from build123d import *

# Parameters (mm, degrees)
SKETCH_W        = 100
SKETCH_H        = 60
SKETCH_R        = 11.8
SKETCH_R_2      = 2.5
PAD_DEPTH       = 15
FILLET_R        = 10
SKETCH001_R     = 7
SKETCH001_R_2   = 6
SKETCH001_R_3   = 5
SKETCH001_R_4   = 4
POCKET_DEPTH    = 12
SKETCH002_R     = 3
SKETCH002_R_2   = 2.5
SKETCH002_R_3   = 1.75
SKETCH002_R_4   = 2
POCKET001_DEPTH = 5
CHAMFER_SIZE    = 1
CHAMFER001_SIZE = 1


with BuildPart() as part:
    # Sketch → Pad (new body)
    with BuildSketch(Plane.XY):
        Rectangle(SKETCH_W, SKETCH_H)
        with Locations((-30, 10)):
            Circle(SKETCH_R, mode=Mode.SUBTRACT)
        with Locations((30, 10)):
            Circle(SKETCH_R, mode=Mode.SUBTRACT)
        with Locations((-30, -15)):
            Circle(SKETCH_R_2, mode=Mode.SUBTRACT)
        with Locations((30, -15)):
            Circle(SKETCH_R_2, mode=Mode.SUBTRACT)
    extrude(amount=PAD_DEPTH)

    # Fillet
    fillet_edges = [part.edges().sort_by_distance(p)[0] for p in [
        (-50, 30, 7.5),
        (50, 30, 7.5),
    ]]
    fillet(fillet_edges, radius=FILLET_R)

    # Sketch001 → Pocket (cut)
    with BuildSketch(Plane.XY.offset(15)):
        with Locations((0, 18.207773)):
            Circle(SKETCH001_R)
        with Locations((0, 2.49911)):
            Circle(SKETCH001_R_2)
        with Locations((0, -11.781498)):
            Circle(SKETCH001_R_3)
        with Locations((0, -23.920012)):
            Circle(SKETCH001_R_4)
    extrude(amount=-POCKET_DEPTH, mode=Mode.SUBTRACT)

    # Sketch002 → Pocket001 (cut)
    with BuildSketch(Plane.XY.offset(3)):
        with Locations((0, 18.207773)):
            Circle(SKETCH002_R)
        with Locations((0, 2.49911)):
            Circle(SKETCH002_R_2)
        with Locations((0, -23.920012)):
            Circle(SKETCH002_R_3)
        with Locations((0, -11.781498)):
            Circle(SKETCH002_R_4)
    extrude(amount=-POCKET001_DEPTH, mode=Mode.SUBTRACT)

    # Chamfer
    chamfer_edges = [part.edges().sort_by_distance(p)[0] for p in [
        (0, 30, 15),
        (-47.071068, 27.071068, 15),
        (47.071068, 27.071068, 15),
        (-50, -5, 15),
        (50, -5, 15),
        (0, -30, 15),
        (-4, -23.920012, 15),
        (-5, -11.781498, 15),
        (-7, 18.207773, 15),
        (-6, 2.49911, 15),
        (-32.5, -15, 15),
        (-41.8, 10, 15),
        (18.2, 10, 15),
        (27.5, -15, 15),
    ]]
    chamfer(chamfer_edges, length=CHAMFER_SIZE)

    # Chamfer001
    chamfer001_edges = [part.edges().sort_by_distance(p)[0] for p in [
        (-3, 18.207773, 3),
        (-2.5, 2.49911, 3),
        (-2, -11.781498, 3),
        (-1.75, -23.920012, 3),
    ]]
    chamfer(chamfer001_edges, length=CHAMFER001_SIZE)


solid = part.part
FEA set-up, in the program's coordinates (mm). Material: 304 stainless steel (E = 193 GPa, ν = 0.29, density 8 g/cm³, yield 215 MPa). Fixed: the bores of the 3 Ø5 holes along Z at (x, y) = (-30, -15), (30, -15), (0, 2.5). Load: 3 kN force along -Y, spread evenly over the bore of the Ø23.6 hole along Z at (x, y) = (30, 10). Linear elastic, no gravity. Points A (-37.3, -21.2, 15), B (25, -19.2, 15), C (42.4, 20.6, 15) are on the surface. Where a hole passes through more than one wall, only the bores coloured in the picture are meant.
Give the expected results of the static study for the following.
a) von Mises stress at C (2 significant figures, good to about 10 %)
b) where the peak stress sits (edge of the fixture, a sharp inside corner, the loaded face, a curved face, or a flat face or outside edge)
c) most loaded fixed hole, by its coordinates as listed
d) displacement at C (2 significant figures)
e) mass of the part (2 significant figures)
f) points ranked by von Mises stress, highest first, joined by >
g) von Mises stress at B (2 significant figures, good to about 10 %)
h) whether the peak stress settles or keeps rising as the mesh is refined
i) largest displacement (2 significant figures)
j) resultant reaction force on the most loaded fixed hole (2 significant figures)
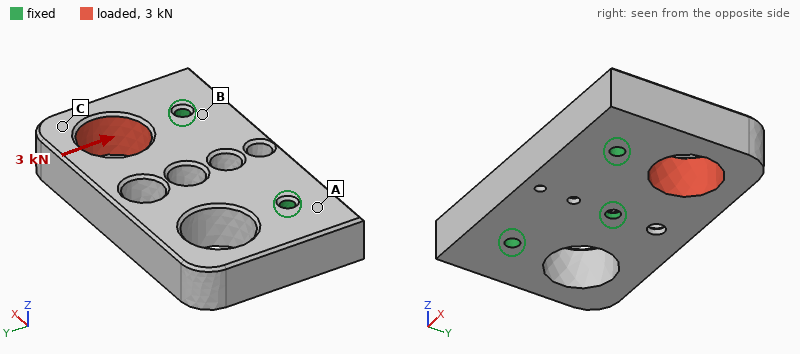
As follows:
4.1 MPa
edge of the fixture
(30, -15)
2.6 µm
560 g
B > C > A
5.8 MPa
keeps rising
3.1 µm
2.7 kN
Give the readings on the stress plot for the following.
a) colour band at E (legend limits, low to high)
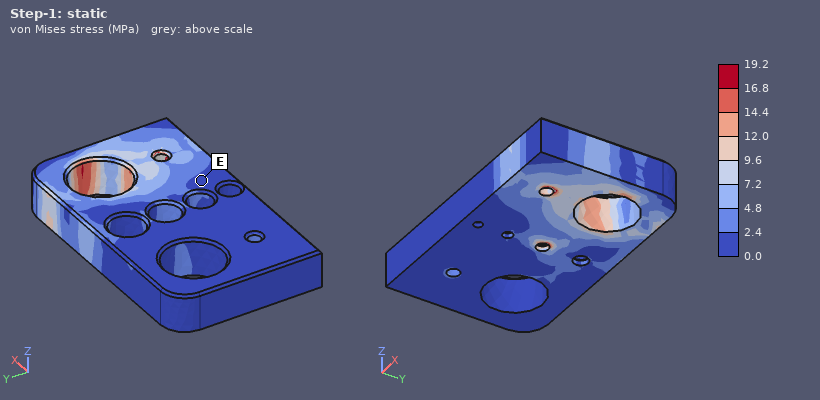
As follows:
0.0 to 2.4 MPa
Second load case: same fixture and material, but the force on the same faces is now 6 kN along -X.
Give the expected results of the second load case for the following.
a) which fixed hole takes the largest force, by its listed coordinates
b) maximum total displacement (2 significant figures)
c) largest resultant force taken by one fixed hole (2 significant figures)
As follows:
(30, -15)
8.2 µm
3.5 kN
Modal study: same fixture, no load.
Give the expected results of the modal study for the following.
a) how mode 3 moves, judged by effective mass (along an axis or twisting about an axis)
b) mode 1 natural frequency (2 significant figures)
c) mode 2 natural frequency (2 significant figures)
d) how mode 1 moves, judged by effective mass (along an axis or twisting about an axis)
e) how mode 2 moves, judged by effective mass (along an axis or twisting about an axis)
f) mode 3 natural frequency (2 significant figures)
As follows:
along X
5100 Hz
5900 Hz
along Z
twisting about Y
9800 Hz
